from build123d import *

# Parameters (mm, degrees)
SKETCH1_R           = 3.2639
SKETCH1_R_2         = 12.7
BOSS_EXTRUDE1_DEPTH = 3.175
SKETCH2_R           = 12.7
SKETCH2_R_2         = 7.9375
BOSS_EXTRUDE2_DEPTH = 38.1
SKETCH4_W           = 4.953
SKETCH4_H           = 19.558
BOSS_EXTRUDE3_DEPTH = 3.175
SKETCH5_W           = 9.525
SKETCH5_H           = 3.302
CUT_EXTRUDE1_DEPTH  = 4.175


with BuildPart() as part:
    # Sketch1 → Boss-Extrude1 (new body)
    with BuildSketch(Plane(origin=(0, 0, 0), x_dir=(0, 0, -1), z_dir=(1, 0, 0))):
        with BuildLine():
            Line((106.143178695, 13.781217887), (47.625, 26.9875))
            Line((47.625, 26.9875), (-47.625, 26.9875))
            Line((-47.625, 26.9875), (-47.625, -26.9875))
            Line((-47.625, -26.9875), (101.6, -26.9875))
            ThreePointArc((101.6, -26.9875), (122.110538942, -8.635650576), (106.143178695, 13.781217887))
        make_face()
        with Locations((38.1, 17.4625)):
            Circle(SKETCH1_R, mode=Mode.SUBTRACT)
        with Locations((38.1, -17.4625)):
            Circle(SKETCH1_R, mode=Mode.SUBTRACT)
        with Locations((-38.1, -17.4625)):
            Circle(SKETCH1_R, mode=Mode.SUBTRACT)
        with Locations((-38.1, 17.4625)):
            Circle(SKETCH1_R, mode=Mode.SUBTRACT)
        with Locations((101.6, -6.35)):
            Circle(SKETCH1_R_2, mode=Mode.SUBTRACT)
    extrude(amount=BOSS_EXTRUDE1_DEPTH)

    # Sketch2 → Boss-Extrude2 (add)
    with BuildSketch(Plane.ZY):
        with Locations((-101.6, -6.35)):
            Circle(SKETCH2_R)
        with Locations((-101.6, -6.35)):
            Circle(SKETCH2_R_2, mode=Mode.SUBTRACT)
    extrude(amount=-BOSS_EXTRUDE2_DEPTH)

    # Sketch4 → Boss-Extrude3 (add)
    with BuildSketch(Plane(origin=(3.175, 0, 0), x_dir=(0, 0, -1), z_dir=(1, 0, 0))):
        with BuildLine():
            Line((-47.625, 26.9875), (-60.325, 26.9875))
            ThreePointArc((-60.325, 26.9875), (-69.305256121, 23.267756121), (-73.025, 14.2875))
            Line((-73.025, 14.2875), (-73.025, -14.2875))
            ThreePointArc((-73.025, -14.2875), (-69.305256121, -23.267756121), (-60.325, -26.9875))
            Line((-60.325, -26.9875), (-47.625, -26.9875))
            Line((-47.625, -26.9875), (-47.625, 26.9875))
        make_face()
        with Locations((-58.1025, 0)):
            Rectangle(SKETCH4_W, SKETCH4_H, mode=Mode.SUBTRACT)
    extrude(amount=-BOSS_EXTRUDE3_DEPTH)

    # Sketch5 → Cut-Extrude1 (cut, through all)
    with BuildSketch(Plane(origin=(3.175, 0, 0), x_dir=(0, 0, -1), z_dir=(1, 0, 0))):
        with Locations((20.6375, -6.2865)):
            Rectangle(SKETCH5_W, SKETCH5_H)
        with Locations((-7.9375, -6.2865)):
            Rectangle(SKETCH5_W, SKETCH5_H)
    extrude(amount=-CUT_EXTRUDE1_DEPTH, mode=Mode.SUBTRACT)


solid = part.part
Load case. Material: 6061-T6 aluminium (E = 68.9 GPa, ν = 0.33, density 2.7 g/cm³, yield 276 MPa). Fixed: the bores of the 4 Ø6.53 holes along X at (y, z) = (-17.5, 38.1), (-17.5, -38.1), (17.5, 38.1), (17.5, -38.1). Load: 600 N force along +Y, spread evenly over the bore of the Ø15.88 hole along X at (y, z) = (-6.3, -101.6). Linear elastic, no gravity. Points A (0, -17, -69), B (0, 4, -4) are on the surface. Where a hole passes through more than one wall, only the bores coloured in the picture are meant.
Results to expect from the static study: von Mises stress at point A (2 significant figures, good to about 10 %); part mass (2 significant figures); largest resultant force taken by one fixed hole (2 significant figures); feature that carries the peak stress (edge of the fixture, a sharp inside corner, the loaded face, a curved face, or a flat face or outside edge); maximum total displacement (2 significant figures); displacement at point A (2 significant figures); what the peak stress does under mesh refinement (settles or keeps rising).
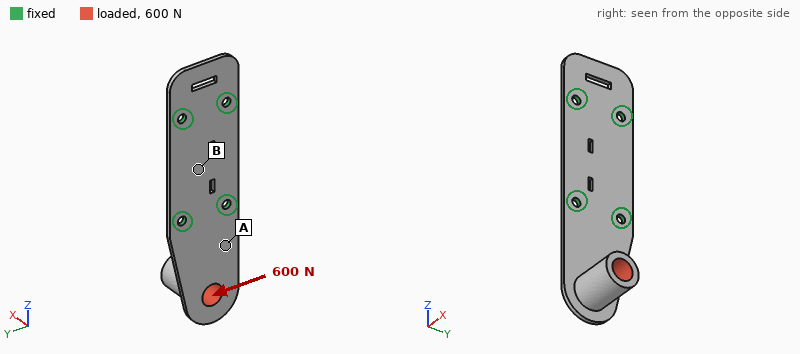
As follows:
90 MPa
110 g
1.0 kN
edge of the fixture
1.2 mm
0.21 mm
keeps rising
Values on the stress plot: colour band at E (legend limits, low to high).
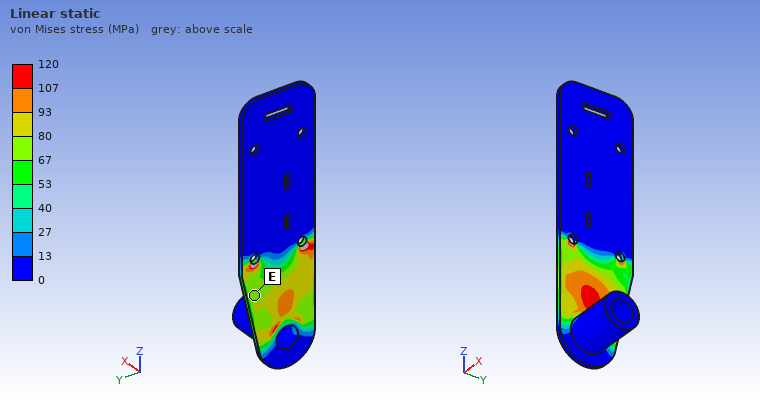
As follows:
67 to 80 MPa
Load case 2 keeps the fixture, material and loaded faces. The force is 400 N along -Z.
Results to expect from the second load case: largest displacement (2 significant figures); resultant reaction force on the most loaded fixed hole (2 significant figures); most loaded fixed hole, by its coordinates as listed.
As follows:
2.4 mm
250 N
(-17.5, -38.1)
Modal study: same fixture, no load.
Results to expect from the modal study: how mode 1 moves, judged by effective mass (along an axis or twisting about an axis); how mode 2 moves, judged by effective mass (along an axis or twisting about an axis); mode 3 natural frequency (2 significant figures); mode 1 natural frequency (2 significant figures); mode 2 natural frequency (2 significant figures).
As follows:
along X
along Y
1300 Hz
250 Hz
710 Hz
